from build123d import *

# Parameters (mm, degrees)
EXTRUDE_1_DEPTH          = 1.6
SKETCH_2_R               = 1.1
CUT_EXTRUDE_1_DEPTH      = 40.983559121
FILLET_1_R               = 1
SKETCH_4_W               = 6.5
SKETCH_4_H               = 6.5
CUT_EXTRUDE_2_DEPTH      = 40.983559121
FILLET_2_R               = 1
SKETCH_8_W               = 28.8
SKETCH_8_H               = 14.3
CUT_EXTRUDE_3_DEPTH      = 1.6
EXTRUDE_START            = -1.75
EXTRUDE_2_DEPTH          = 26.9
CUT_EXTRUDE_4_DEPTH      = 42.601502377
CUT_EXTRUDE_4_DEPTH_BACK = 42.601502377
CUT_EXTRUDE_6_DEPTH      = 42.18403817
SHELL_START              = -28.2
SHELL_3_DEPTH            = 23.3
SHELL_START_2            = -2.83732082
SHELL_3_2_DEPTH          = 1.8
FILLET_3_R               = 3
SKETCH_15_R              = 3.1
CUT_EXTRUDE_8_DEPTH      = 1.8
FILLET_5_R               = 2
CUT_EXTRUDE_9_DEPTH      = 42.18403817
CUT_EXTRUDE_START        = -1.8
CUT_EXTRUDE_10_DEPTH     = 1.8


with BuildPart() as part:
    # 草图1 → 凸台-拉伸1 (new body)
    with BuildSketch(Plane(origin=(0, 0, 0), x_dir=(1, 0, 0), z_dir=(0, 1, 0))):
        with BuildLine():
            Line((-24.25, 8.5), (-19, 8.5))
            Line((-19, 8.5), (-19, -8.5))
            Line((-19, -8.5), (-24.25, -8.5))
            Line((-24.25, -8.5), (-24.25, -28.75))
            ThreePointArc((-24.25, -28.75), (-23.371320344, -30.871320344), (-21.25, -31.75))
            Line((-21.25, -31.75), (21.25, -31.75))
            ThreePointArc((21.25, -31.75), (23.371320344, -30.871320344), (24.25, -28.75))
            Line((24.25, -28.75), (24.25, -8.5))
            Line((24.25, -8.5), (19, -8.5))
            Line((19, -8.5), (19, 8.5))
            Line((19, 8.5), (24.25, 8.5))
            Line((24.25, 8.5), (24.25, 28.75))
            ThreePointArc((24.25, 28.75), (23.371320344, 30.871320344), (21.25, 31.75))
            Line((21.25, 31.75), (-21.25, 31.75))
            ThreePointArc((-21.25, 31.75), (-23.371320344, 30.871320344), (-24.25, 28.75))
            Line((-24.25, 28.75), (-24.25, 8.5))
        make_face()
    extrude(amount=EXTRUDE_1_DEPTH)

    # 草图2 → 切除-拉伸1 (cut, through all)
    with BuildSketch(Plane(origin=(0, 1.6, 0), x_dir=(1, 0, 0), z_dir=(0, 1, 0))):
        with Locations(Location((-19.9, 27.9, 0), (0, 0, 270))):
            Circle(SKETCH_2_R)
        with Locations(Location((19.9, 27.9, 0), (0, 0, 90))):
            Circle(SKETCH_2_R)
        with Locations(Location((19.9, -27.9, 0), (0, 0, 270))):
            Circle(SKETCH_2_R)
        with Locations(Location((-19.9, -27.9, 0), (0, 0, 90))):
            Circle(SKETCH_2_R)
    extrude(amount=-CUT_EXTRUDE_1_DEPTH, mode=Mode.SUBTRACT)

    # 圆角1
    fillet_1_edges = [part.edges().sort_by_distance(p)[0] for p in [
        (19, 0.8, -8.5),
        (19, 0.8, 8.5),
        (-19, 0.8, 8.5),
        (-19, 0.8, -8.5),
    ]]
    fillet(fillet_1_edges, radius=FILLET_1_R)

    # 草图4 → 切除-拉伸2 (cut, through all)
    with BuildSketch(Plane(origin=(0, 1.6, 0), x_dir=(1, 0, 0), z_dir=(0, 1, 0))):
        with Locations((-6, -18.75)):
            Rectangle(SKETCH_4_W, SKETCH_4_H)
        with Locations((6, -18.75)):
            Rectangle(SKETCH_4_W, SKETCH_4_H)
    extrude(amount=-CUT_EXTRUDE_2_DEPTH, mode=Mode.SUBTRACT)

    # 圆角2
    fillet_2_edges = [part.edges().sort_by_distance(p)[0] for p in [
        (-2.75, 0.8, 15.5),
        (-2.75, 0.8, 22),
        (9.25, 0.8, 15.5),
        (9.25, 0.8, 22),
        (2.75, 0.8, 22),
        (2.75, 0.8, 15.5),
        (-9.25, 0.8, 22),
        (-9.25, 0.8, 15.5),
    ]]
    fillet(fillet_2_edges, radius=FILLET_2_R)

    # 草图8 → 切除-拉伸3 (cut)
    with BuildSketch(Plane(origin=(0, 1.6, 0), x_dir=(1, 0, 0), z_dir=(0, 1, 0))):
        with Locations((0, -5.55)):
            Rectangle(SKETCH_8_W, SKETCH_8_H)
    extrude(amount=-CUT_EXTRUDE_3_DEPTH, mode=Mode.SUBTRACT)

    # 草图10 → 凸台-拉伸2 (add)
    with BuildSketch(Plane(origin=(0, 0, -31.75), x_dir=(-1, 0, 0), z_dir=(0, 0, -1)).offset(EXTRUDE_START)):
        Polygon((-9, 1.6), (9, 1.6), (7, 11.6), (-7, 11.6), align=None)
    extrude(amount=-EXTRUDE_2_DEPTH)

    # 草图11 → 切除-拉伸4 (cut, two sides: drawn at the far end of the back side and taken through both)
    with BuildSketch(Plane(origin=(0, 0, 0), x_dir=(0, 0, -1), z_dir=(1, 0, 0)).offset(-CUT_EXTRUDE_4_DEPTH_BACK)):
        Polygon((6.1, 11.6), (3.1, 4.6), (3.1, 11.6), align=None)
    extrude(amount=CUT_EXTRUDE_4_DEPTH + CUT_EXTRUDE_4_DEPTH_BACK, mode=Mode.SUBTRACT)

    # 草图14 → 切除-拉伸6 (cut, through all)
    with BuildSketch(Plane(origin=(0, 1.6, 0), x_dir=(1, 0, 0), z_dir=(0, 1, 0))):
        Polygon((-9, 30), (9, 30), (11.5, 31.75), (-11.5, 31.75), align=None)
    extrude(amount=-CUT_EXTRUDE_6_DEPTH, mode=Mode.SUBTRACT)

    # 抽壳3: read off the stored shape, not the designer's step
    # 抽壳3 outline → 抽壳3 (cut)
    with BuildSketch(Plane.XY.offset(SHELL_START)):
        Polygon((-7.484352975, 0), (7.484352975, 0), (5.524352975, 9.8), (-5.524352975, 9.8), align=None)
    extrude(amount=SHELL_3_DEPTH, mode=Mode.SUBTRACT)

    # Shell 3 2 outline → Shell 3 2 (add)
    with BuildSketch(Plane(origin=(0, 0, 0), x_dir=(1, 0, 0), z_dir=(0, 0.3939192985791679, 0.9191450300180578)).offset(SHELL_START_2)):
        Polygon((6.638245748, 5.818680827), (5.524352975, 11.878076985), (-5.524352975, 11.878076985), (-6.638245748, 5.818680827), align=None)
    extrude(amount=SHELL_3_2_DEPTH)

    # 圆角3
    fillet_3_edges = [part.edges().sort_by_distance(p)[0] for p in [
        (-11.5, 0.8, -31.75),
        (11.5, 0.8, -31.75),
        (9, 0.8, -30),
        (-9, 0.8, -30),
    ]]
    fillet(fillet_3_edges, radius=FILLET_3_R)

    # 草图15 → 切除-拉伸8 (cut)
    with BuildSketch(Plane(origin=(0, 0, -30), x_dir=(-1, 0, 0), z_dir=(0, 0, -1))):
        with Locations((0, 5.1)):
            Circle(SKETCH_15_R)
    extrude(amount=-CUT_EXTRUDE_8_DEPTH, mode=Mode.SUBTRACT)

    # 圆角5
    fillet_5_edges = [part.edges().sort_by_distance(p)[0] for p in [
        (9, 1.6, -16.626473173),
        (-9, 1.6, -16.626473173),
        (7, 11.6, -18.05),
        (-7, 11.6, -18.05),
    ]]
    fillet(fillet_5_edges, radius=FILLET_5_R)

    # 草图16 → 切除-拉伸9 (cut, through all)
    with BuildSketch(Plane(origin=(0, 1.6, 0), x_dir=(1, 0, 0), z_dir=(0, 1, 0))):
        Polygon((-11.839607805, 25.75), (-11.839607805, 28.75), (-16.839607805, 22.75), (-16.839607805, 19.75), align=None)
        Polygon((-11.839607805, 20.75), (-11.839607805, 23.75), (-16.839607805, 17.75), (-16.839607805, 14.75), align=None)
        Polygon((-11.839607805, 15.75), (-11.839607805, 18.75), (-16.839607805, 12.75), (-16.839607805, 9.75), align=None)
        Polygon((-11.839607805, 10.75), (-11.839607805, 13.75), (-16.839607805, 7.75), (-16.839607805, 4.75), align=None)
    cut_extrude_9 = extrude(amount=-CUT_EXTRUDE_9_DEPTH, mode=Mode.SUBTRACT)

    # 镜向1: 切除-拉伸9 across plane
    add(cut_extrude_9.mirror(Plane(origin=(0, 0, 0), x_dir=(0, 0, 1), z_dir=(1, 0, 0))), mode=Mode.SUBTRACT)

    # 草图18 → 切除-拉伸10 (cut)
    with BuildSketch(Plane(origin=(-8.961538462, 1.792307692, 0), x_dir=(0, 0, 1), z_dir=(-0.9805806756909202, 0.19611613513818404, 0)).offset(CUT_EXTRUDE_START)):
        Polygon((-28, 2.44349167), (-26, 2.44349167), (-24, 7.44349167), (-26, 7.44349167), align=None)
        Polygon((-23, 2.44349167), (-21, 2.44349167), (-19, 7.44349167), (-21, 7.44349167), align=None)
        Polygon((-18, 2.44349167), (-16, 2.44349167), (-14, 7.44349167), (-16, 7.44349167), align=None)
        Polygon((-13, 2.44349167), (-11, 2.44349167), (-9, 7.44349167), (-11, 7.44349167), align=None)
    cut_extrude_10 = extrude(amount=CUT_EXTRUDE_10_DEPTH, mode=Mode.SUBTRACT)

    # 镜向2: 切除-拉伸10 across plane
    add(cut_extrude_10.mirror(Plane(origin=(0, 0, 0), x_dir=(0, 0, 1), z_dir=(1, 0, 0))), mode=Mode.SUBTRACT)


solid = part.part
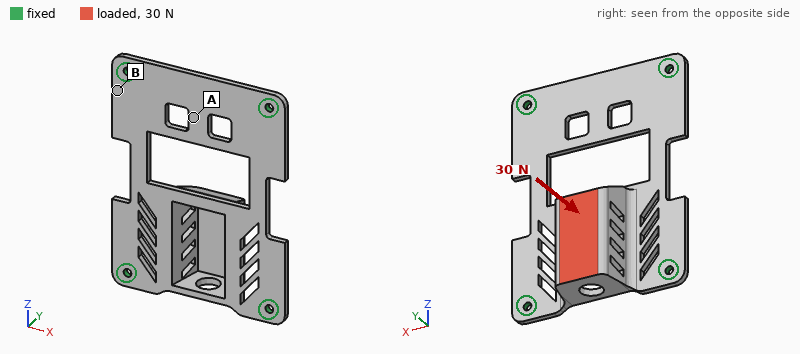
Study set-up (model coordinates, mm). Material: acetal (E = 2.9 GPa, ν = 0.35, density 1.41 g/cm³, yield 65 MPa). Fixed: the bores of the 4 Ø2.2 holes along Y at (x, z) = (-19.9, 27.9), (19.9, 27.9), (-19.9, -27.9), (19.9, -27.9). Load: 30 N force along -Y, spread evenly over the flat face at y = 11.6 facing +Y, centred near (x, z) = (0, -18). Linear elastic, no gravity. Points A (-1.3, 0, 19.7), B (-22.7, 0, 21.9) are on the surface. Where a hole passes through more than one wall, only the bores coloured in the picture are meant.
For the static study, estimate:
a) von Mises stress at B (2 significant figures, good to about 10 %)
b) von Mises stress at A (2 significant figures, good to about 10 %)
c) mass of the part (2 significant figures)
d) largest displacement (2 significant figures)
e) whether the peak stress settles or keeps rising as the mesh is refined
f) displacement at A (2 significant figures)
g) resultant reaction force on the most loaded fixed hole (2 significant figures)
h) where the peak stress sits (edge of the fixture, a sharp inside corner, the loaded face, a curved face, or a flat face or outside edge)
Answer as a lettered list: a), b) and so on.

a) 5.5 MPa
b) 1.7 MPa
c) 6.5 g
d) 0.80 mm
e) keeps rising
f) 0.15 mm
g) 14 N
h) edge of the fixture
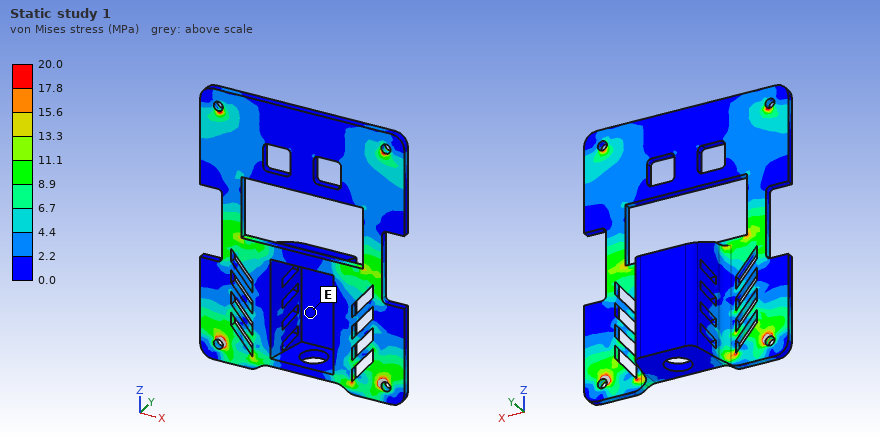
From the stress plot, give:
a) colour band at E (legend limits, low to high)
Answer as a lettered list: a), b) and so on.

a) 0.0 to 2.2 MPa
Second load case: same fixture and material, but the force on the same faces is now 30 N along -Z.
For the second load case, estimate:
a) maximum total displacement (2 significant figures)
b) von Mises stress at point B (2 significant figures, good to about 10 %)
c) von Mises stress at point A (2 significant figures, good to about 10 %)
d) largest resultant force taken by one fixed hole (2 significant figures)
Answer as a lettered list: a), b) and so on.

a) 0.83 mm
b) 6.3 MPa
c) 1.8 MPa
d) 11 N
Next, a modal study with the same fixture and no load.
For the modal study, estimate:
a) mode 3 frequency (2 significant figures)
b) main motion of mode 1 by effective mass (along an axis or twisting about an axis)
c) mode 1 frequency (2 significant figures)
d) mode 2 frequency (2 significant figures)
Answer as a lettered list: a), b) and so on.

a) 1300 Hz
b) along Y
c) 480 Hz
d) 1200 Hz
